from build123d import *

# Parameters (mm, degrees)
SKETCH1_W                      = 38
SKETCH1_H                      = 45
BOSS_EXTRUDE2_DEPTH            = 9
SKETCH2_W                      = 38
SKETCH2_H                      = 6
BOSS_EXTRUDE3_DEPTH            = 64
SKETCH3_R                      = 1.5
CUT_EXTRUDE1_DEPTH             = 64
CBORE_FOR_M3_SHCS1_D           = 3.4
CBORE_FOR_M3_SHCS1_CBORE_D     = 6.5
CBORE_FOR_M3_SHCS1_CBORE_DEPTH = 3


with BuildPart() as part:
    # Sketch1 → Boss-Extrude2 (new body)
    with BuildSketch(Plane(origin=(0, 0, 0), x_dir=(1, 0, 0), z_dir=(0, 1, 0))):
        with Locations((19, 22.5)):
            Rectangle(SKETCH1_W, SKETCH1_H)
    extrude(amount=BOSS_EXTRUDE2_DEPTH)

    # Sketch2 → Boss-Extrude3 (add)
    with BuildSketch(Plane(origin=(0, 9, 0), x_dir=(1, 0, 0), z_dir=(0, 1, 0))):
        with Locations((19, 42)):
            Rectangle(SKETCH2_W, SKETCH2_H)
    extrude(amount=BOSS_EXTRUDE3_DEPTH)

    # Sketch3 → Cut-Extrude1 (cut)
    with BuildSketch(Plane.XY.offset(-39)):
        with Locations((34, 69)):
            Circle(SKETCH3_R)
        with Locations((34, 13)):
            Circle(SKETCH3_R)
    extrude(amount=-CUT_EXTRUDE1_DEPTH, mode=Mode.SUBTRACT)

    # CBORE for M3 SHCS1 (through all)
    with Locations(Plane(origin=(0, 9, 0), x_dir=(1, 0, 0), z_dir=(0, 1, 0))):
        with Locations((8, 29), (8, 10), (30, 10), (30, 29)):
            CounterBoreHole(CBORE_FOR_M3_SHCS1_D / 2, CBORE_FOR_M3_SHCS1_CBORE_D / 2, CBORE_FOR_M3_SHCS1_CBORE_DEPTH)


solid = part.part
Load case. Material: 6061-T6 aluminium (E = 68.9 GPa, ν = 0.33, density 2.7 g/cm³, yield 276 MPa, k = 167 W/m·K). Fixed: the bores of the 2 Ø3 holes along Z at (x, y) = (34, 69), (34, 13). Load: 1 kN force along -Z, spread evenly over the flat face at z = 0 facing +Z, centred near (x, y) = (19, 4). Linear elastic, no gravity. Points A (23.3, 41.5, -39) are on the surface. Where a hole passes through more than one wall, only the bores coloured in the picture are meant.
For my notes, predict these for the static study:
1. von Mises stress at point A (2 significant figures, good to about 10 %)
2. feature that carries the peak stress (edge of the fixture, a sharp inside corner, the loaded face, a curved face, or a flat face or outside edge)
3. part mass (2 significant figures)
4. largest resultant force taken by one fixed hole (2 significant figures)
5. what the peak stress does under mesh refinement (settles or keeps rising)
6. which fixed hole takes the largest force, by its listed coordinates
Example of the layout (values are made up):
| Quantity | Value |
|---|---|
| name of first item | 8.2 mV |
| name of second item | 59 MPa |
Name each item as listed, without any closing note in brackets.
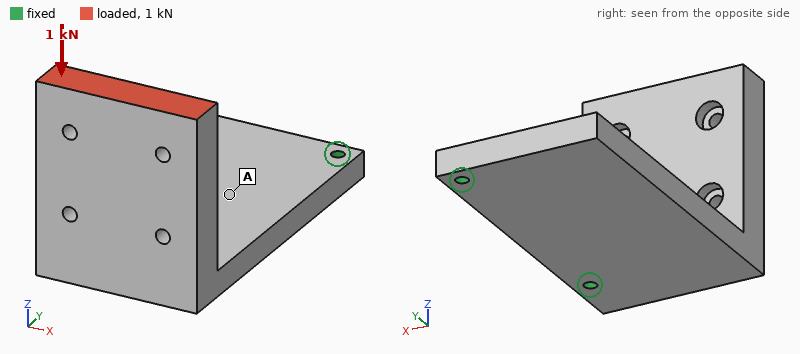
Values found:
| Quantity | Value |
|---|---|
| von Mises stress at point A | 13 MPa |
| feature that carries the peak stress | edge of the fixture |
| part mass | 79 g |
| largest resultant force taken by one fixed hole | 1.1 kN |
| what the peak stress does under mesh refinement | keeps rising |
| which fixed hole takes the largest force, by its listed coordinates | (34, 13) |
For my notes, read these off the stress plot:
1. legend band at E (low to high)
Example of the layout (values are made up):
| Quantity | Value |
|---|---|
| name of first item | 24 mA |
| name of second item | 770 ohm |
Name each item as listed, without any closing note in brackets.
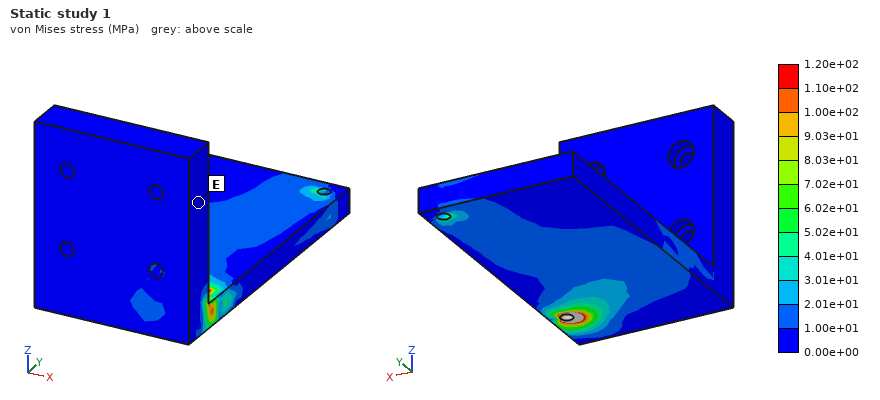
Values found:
| Quantity | Value |
|---|---|
| legend band at E | 0.00e+00 to 1.00e+01 MPa |
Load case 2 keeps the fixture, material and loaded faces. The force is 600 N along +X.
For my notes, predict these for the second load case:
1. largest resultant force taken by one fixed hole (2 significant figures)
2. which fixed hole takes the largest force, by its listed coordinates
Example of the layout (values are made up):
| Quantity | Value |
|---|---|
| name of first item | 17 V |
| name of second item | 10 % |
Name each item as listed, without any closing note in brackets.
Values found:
| Quantity | Value |
|---|---|
| largest resultant force taken by one fixed hole | 680 N |
| which fixed hole takes the largest force, by its listed coordinates | (34, 13) |
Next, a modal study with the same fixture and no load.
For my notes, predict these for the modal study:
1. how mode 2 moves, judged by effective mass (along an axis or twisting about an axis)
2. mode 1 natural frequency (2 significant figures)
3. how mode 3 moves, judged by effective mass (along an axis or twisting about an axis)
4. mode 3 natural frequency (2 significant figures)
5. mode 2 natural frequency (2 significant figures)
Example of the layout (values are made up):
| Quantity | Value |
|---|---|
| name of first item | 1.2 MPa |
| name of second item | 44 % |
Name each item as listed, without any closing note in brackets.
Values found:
| Quantity | Value |
|---|---|
| how mode 2 moves, judged by effective mass | along Y |
| mode 1 natural frequency | 1500 Hz |
| how mode 3 moves, judged by effective mass | along Z |
| mode 3 natural frequency | 4100 Hz |
| mode 2 natural frequency | 1900 Hz |
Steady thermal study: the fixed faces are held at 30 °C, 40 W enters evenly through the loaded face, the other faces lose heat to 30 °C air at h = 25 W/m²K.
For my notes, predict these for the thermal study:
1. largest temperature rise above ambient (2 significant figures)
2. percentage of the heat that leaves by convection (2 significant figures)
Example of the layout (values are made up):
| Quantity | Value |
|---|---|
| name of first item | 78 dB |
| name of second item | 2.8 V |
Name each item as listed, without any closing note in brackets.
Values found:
| Quantity | Value |
|---|---|
| largest temperature rise above ambient | 47 K |
| percentage of the heat that leaves by convection | 11 % |
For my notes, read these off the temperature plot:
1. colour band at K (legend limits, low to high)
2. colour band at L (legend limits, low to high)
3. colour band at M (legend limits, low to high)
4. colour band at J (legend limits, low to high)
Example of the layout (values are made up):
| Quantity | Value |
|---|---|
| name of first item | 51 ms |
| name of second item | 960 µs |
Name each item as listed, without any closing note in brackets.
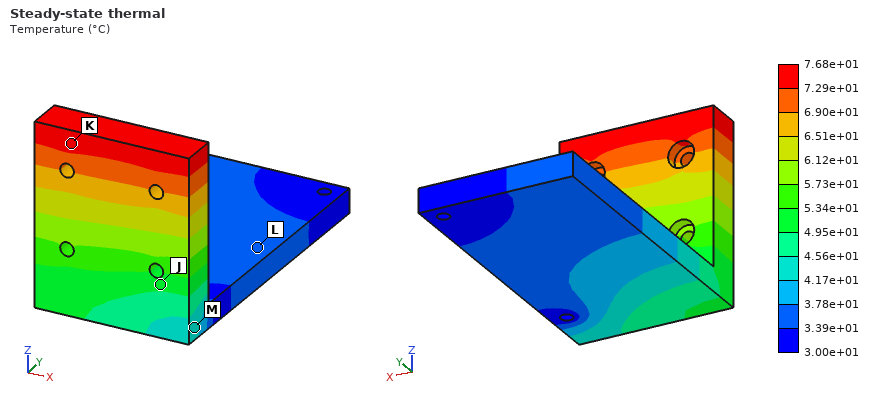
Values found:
| Quantity | Value |
|---|---|
| colour band at K | 7.29e+01 to 7.68e+01 °C |
| colour band at L | 3.39e+01 to 3.78e+01 °C |
| colour band at M | 4.17e+01 to 4.56e+01 °C |
| colour band at J | 4.95e+01 to 5.34e+01 °C |
